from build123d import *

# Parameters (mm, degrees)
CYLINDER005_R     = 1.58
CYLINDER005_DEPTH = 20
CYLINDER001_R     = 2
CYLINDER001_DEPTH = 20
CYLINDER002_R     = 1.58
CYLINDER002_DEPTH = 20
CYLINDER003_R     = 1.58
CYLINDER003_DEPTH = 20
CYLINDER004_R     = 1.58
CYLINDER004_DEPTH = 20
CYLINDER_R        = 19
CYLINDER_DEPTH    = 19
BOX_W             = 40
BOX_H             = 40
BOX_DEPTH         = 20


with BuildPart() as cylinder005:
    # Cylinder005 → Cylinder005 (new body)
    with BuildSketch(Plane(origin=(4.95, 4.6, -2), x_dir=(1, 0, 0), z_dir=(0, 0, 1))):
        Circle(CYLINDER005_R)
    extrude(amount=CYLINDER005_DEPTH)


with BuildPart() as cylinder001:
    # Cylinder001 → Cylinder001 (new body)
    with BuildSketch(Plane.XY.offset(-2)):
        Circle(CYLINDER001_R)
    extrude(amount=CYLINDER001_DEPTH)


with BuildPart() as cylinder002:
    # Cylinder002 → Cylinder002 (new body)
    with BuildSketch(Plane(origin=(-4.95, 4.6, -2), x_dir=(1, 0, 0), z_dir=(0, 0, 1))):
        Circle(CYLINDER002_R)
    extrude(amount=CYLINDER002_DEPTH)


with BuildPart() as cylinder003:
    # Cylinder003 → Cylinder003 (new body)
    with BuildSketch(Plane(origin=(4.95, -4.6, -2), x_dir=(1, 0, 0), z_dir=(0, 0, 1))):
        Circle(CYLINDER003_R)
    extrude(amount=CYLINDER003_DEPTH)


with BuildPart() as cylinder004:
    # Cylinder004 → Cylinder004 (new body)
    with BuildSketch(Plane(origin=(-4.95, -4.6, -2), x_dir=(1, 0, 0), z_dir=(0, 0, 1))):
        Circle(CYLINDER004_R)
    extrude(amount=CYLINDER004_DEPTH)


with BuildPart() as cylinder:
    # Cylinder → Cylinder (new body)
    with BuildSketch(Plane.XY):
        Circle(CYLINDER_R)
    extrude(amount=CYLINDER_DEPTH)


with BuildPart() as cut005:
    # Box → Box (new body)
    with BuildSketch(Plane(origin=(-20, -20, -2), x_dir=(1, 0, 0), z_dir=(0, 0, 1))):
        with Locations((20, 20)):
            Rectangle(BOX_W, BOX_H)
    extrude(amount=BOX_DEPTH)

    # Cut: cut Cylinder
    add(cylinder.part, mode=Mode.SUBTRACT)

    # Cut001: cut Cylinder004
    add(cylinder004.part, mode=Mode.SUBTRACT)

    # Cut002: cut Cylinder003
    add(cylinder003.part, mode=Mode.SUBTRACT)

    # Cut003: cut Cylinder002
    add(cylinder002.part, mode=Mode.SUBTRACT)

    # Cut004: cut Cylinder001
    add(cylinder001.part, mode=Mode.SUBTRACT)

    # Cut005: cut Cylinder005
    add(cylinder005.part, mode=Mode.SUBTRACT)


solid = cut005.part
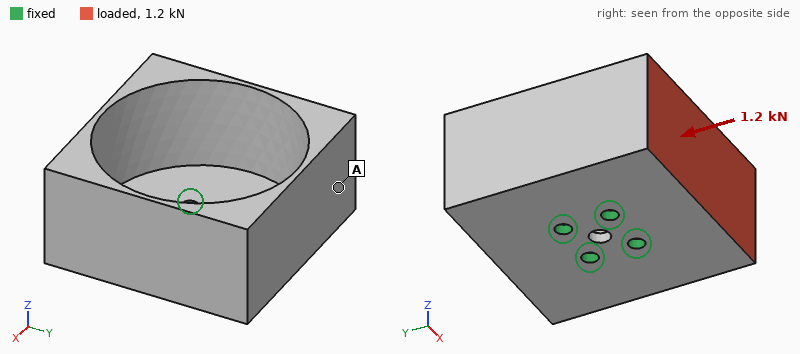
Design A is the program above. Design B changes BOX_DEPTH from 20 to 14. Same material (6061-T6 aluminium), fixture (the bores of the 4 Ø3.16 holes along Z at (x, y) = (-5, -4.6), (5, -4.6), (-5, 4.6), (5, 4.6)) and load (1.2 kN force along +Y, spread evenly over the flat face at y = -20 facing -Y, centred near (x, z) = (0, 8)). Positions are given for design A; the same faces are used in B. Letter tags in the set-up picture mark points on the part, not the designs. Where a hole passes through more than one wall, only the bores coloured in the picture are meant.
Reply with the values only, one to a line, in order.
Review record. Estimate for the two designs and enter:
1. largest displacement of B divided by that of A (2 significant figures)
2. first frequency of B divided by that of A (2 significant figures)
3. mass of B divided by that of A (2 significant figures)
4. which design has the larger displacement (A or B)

0.69
1.3
0.76
A
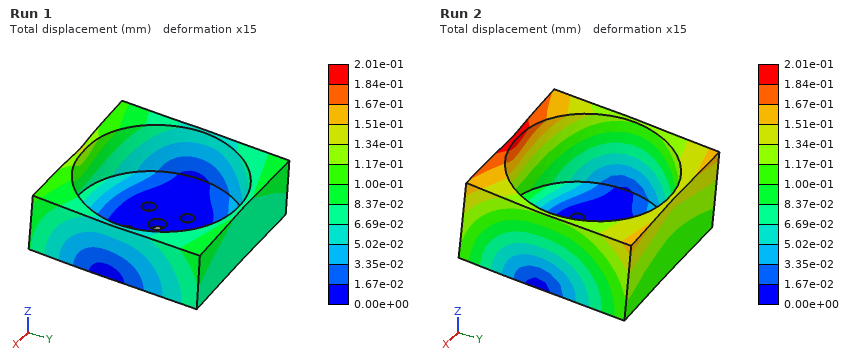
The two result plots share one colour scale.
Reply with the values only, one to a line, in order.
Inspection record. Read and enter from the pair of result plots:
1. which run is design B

Run 1
